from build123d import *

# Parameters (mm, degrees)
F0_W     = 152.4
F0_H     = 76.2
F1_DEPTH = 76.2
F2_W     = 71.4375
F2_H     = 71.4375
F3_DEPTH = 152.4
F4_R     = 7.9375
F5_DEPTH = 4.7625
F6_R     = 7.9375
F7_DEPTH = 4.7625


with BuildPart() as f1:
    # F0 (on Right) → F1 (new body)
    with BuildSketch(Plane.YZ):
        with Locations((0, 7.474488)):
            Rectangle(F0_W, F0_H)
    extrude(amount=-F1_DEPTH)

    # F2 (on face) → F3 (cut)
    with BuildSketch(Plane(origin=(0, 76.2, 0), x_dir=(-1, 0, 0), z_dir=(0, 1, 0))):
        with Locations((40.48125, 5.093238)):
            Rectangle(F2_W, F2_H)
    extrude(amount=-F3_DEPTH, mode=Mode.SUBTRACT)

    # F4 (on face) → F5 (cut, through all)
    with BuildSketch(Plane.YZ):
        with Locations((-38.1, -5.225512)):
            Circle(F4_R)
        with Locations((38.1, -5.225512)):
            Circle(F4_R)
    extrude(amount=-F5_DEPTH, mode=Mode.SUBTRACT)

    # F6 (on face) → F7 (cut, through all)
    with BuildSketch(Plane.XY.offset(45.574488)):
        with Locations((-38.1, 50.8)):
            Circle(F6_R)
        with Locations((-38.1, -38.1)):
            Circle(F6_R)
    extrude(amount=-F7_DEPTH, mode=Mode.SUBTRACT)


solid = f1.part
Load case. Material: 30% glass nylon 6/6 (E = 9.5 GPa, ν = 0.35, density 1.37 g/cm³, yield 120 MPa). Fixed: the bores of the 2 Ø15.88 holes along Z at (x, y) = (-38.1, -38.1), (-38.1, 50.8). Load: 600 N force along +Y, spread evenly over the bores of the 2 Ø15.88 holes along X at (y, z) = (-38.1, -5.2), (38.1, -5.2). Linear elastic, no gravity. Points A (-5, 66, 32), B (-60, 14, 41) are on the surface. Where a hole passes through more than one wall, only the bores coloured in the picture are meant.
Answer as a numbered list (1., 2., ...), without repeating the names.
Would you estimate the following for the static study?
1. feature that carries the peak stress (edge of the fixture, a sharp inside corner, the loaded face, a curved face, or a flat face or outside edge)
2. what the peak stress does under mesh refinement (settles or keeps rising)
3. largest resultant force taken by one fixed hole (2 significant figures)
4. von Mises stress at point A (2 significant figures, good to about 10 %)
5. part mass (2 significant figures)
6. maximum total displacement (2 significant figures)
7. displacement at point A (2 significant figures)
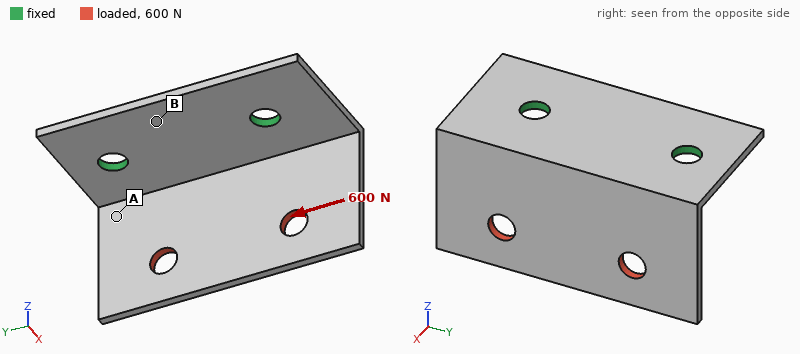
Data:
1. edge of the fixture
2. keeps rising
3. 470 N
4. 10 MPa
5. 140 g
6. 1.2 mm
7. 0.49 mm
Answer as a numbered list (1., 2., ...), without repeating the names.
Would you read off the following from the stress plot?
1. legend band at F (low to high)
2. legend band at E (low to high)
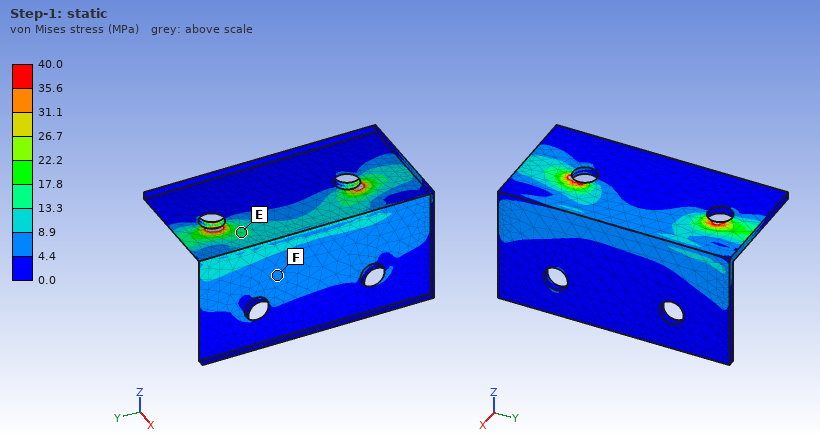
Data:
1. 4.4 to 8.9 MPa
2. 13.3 to 17.8 MPa
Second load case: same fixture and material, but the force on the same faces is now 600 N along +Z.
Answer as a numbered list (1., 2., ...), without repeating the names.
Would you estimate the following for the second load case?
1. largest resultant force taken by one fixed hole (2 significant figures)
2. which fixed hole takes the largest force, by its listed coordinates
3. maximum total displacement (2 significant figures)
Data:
1. 340 N
2. (-38.1, -38.1)
3. 1.9 mm
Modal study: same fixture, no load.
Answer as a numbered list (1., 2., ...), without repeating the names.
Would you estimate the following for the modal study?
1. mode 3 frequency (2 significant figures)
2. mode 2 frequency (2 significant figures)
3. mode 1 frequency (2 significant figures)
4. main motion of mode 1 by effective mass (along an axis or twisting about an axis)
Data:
1. 710 Hz
2. 410 Hz
3. 230 Hz
4. along X
